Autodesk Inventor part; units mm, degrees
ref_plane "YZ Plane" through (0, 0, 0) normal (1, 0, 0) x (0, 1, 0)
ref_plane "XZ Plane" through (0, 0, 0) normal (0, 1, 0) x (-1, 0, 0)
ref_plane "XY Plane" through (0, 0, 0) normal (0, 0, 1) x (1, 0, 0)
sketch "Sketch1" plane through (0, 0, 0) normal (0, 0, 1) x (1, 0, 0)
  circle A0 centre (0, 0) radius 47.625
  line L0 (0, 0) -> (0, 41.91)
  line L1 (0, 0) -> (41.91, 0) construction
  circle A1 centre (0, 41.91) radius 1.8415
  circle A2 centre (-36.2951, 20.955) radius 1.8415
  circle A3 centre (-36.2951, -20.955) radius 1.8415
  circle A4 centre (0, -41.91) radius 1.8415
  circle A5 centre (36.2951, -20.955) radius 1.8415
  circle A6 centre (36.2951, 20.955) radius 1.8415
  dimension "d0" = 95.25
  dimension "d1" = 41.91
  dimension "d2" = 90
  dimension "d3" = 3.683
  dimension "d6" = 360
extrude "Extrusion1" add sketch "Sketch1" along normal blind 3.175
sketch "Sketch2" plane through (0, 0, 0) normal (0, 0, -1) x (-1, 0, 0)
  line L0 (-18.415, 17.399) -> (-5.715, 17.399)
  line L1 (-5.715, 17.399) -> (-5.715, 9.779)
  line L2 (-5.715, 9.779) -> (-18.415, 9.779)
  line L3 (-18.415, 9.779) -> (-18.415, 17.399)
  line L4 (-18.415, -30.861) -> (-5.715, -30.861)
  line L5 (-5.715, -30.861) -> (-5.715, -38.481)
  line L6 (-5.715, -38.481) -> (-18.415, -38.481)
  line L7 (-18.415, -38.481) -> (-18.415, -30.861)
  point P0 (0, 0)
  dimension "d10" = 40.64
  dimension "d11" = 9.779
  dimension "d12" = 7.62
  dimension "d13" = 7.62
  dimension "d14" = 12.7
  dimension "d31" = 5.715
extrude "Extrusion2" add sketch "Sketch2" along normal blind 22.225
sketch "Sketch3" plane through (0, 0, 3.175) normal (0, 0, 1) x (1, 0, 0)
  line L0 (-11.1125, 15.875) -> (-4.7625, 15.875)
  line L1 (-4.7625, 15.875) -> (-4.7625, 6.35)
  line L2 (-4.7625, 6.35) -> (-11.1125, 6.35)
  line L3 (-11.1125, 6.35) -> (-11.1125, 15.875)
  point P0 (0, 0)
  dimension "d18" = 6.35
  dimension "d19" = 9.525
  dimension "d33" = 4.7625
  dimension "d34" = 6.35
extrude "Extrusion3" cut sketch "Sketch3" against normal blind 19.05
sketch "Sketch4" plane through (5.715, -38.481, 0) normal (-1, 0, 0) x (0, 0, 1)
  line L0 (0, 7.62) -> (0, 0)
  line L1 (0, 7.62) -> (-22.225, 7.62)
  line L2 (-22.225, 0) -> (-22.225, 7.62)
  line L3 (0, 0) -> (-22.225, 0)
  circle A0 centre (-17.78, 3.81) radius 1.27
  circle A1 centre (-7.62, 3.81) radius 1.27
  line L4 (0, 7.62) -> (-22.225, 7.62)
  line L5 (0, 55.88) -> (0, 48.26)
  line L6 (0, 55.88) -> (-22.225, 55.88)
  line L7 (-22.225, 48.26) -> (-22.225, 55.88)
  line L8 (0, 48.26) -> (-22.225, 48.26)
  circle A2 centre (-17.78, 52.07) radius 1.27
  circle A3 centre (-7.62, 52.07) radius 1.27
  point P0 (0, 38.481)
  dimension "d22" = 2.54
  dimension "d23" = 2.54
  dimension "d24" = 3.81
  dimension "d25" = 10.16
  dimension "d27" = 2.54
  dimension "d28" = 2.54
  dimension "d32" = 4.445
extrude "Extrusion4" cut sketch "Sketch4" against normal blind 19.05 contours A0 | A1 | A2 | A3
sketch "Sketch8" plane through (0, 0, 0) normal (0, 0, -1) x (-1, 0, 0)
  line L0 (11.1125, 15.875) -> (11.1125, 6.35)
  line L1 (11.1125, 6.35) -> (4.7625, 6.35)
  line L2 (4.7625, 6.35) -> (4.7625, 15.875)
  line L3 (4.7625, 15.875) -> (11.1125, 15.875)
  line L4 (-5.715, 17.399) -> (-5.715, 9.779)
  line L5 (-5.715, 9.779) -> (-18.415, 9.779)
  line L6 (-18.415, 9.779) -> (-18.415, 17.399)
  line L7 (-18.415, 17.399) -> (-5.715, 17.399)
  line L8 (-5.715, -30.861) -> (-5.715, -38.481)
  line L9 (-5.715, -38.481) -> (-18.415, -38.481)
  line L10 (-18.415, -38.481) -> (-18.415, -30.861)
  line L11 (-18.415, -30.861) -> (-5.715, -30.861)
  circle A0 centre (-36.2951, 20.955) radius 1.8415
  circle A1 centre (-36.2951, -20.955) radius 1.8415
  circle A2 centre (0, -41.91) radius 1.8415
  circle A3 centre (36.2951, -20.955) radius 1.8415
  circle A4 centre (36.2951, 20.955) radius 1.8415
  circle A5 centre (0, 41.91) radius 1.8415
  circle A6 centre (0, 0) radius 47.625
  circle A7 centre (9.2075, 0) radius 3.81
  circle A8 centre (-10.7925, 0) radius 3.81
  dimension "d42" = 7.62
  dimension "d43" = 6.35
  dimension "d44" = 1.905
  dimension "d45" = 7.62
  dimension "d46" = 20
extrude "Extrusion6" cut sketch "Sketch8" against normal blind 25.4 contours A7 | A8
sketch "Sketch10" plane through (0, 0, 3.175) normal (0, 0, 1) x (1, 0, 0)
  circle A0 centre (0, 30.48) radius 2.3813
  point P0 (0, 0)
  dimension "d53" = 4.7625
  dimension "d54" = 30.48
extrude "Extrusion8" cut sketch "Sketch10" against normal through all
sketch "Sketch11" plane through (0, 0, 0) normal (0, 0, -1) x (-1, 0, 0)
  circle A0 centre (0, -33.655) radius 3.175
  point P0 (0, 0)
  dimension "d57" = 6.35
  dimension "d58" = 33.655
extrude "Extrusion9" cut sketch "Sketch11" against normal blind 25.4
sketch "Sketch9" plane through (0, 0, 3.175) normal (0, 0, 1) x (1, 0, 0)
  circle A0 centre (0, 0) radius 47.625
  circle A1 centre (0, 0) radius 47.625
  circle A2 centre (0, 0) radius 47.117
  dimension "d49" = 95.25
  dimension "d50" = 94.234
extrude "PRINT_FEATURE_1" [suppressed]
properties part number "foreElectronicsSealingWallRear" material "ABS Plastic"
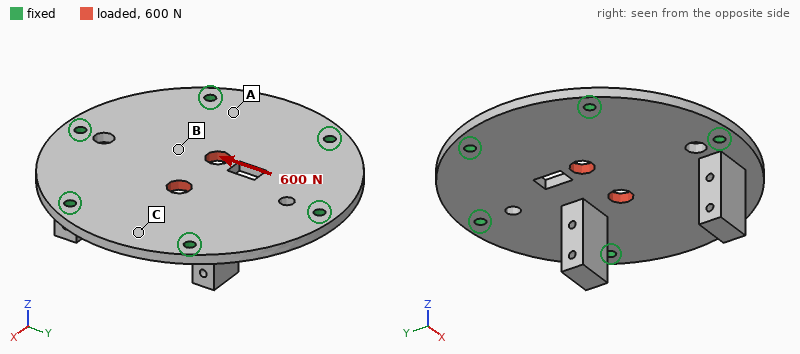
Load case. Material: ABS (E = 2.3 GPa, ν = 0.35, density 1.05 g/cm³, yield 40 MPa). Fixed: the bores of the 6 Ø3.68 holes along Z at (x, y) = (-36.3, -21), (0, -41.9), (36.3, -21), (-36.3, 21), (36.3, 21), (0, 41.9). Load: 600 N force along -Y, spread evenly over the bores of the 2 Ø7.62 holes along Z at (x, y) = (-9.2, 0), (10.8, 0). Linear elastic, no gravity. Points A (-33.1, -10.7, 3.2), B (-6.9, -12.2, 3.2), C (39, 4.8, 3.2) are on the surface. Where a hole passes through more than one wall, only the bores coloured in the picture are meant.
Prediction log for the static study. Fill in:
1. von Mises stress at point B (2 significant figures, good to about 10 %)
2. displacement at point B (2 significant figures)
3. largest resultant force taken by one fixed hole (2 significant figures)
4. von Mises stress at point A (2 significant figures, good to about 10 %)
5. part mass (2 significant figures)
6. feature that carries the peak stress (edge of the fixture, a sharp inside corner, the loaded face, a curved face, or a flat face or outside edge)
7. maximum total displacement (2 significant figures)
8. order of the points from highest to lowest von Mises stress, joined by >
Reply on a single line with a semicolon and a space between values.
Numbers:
2.3 MPa; 37 µm; 130 N; 1.3 MPa; 27 g; a flat face or outside edge; 62 µm; B > A > C
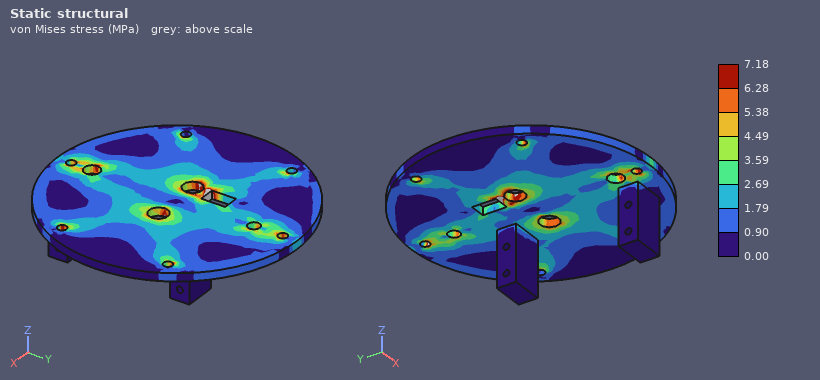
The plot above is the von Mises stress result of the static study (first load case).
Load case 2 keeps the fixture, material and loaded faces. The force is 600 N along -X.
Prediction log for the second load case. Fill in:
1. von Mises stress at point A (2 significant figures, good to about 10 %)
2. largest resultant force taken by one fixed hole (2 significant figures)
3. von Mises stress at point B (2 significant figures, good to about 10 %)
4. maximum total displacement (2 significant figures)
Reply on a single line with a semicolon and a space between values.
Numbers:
1.9 MPa; 140 N; 1.7 MPa; 61 µm
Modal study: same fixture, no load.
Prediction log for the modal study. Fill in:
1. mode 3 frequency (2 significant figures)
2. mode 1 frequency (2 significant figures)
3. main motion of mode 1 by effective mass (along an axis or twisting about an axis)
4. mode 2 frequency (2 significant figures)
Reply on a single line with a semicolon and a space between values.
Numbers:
1500 Hz; 890 Hz; along Z; 1400 Hz
